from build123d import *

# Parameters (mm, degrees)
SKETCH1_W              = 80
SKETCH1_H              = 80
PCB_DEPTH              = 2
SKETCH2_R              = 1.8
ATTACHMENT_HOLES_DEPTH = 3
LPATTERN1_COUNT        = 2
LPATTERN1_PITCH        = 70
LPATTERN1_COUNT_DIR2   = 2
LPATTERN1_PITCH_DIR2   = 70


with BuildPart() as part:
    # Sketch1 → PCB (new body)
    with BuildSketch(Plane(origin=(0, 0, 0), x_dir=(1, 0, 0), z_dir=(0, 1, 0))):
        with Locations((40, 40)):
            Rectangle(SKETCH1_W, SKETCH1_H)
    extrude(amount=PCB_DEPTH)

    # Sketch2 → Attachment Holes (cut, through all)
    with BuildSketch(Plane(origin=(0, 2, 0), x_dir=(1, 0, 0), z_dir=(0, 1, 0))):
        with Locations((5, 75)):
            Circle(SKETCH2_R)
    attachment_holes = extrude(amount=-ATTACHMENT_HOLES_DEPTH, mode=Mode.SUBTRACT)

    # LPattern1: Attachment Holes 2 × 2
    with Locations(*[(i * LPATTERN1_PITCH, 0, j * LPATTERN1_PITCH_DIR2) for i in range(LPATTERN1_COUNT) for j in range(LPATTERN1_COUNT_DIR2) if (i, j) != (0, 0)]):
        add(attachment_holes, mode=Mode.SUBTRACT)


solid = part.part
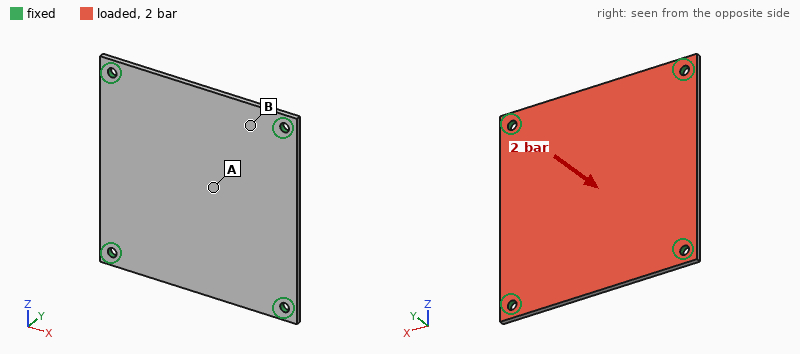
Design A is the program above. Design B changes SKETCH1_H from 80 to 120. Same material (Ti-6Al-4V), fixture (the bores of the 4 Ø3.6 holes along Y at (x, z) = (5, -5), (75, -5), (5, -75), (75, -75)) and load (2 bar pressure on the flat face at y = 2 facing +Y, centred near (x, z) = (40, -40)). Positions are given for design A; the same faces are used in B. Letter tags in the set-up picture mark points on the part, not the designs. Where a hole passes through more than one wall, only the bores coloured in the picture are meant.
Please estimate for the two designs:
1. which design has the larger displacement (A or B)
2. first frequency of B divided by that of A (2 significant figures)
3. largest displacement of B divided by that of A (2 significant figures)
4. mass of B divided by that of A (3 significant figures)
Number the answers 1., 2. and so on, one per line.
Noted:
1. A
2. 1.0
3. 0.85
4. 1.50
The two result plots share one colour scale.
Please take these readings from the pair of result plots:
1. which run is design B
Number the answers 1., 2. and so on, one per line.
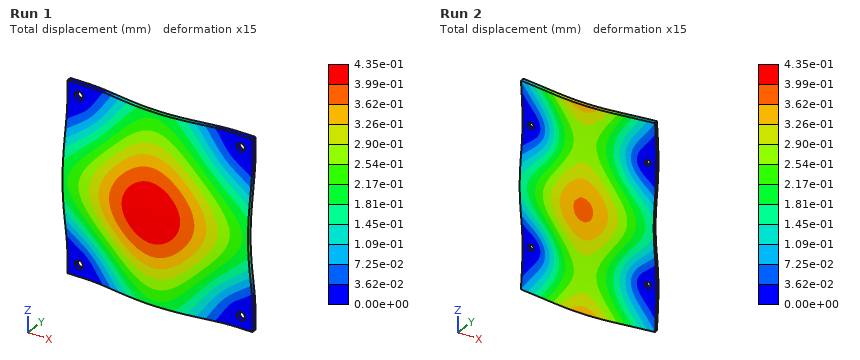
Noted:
1. Run 2
